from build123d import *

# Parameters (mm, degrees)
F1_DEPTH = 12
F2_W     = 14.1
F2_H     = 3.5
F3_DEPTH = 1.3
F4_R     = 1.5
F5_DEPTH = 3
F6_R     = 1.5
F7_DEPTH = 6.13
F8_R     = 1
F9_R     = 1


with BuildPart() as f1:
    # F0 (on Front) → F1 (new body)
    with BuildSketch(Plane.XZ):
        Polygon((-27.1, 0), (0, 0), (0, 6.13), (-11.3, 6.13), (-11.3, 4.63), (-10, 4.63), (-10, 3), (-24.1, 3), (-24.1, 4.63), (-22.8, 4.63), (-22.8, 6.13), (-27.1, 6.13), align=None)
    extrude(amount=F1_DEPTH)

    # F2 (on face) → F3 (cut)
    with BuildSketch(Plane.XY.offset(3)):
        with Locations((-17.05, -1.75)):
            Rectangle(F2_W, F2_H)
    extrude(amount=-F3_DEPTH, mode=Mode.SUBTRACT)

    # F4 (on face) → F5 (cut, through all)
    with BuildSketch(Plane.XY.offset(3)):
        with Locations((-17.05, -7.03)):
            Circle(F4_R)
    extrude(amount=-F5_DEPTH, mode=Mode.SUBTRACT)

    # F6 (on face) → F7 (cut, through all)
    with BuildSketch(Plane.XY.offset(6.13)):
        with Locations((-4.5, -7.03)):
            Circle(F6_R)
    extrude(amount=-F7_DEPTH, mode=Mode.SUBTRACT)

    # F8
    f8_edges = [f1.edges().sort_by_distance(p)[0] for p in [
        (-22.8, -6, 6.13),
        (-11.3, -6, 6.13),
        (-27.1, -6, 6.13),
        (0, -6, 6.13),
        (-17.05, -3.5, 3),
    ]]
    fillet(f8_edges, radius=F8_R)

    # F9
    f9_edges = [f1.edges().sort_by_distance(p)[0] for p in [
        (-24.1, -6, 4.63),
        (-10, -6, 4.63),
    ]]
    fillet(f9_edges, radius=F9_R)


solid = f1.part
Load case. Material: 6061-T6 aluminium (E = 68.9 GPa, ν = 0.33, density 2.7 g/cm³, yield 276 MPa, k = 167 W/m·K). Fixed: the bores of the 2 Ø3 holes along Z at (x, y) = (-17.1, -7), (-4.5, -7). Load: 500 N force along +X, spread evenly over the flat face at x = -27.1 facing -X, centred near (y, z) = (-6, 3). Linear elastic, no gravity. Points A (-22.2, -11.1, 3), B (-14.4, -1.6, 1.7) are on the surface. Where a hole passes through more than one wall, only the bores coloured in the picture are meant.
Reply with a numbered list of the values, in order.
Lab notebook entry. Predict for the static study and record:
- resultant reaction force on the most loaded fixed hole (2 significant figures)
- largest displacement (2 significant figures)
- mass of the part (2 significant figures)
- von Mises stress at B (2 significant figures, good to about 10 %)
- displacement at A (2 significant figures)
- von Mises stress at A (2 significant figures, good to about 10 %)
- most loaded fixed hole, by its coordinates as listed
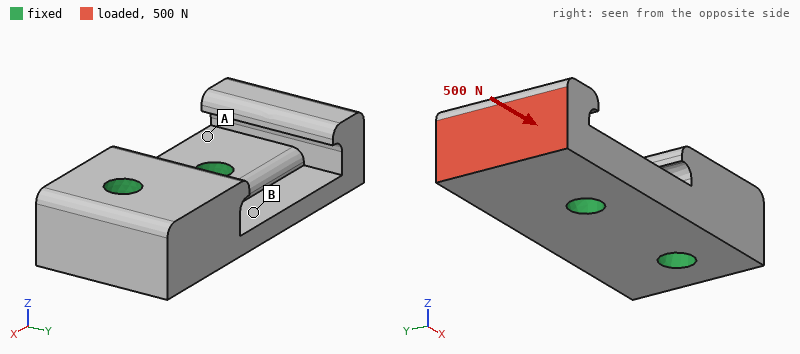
1. 450 N
2. 28 µm
3. 3.7 g
4. 9.9 MPa
5. 5.1 µm
6. 44 MPa
7. (-17.1, -7)
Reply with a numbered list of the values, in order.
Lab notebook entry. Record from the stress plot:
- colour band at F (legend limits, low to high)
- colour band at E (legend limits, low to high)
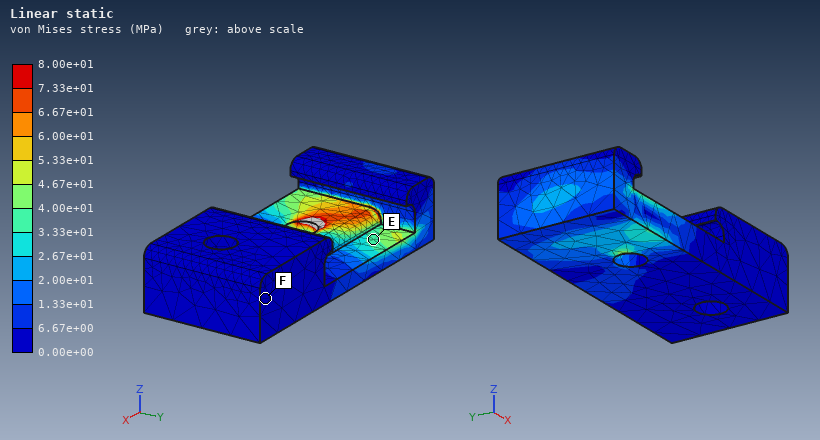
1. 0.00e+00 to 6.67e+00 MPa
2. 3.33e+01 to 4.00e+01 MPa
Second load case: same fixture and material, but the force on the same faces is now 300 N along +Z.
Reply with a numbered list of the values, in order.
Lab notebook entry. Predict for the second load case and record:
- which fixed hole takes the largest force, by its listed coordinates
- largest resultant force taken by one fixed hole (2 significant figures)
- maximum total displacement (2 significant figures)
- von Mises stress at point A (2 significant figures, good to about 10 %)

1. (-17.1, -7)
2. 350 N
3. 81 µm
4. 91 MPa
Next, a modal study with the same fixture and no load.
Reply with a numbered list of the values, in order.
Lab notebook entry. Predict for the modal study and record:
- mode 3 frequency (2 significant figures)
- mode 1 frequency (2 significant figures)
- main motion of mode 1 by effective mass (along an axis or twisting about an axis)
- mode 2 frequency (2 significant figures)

1. 33 kHz
2. 15 kHz
3. along Z
4. 22 kHz
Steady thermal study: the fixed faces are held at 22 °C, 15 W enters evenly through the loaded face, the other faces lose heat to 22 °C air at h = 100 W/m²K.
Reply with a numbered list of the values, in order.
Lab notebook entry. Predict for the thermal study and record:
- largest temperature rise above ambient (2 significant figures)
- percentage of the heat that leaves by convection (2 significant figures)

1. 27 K
2. 4.5 %
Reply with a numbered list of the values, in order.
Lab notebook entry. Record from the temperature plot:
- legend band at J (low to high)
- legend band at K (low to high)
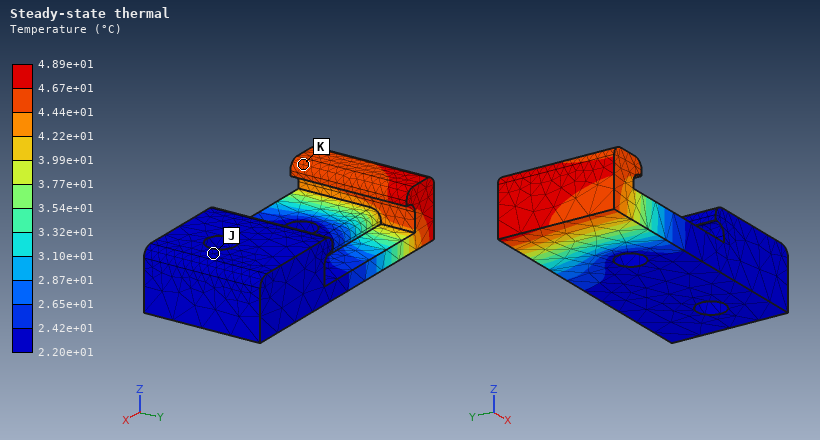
1. 2.20e+01 to 2.42e+01 °C
2. 4.44e+01 to 4.67e+01 °C
